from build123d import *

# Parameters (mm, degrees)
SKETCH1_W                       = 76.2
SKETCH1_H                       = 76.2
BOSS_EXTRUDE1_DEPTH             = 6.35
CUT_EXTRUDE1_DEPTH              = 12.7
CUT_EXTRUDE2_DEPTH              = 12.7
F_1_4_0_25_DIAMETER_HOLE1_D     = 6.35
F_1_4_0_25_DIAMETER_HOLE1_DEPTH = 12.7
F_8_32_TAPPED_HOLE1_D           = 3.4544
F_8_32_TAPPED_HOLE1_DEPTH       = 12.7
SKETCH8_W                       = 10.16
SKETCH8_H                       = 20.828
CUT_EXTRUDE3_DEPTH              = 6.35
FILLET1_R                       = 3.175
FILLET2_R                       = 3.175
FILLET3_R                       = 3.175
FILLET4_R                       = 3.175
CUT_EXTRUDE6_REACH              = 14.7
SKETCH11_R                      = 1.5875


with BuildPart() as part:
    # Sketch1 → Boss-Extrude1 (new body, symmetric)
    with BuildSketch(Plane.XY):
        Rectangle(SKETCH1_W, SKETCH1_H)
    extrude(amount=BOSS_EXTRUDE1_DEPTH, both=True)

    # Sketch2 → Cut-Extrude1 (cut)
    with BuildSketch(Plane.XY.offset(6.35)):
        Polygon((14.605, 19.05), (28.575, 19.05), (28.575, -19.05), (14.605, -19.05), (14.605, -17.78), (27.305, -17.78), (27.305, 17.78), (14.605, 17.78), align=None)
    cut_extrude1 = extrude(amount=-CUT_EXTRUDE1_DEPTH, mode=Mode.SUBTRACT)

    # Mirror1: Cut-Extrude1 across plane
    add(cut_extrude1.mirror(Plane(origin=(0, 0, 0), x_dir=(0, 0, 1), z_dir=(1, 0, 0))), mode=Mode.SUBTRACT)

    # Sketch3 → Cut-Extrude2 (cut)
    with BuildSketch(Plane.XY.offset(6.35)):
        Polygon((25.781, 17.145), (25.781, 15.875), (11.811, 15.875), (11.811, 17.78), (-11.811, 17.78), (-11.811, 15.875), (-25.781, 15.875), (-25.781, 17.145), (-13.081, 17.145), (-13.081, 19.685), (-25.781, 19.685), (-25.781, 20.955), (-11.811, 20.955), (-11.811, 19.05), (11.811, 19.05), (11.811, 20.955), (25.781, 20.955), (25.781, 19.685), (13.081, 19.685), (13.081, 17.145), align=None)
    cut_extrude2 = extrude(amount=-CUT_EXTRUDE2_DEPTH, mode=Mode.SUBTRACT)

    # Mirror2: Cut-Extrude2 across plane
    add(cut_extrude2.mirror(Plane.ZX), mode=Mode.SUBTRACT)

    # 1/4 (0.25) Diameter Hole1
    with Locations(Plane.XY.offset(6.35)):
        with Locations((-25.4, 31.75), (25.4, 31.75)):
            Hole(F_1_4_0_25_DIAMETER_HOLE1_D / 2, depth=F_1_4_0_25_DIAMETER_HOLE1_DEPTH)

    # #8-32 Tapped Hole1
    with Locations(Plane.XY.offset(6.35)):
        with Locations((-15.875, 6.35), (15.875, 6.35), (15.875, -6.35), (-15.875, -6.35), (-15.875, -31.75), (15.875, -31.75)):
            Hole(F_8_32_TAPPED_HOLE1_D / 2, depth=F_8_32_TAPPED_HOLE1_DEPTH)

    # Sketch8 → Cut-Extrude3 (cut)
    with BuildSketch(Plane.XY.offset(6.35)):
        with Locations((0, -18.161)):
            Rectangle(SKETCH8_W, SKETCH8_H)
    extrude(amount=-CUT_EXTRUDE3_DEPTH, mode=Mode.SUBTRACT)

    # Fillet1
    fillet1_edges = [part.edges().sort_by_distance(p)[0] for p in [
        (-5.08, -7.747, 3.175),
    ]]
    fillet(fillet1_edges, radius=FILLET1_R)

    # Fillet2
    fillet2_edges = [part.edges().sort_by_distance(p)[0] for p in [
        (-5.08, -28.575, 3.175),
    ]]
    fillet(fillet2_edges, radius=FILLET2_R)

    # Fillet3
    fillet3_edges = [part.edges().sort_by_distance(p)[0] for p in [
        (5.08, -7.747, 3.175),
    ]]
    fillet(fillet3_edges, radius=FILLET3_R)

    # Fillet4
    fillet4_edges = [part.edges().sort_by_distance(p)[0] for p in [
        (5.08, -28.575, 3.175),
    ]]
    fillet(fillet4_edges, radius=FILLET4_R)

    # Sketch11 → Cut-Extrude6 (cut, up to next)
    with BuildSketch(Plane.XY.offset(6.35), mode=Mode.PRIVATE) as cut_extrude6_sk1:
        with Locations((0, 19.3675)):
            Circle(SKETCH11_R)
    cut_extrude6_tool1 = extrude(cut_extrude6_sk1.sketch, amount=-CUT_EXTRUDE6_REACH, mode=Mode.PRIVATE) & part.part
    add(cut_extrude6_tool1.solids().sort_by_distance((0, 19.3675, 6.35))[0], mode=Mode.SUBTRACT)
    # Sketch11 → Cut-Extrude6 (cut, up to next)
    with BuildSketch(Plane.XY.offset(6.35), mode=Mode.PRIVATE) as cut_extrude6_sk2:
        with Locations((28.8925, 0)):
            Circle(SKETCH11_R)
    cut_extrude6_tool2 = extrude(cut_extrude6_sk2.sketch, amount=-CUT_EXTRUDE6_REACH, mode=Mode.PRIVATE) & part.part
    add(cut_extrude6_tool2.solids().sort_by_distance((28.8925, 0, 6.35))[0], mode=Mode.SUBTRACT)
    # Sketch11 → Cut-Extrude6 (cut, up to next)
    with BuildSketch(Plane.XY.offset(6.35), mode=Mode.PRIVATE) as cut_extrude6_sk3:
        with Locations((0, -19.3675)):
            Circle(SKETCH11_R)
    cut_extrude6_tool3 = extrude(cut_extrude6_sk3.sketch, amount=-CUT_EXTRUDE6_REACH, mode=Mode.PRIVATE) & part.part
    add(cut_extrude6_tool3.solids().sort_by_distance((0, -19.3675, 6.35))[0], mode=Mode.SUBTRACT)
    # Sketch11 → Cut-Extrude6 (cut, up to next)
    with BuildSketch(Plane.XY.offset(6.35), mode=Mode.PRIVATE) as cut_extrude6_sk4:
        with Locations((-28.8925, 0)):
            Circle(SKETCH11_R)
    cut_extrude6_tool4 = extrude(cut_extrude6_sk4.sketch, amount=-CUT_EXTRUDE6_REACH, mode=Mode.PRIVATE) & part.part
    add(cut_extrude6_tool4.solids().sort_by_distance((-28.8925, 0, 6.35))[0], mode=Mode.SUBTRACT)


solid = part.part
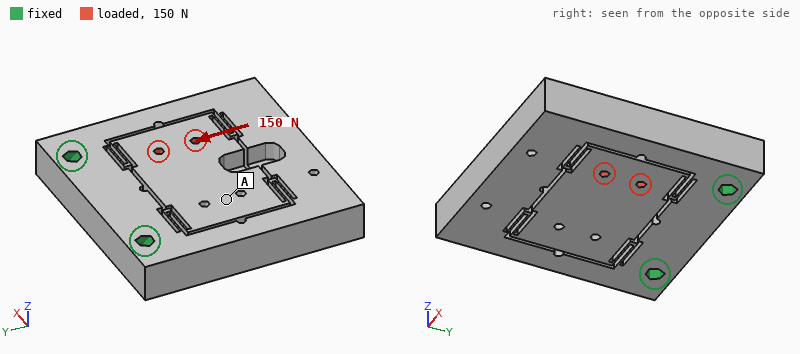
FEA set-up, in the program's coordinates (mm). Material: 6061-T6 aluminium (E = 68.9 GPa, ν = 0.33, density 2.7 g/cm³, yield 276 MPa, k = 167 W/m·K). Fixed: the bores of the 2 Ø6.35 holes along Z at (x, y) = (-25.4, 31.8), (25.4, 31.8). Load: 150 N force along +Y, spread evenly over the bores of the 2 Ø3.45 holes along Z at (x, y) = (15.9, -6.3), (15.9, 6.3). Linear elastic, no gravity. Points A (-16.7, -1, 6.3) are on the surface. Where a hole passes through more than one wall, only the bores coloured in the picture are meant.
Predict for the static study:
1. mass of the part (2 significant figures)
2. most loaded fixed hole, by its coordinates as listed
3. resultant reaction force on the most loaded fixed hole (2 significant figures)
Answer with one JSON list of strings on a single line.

["180 g", "(25.4, 31.8)", "110 N"]
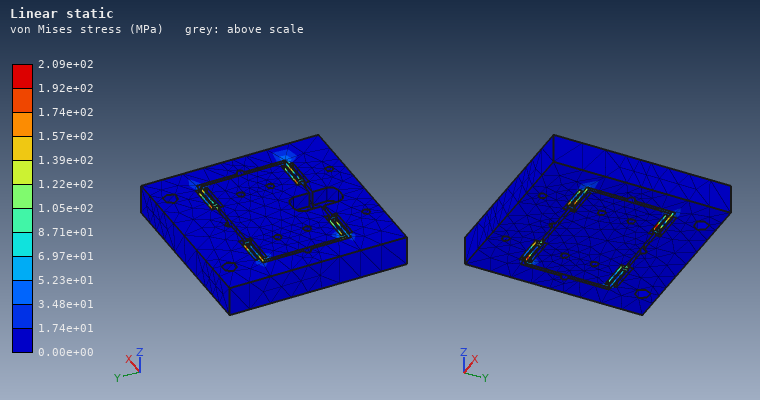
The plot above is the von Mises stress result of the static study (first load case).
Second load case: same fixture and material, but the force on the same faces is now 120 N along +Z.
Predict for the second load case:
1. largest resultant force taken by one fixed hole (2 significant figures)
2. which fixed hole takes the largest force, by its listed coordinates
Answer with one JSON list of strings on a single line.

["95 N", "(25.4, 31.8)"]
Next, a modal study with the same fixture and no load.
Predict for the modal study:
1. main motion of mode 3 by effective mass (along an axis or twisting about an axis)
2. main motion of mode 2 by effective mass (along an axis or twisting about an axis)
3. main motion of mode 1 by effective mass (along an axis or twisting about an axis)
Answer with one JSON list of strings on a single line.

["along X", "along Z", "along Y"]
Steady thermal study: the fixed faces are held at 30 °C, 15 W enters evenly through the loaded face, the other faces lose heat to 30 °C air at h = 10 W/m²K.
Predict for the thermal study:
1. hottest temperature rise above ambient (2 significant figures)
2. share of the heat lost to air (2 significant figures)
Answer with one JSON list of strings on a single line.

["60 K", "33 %"]
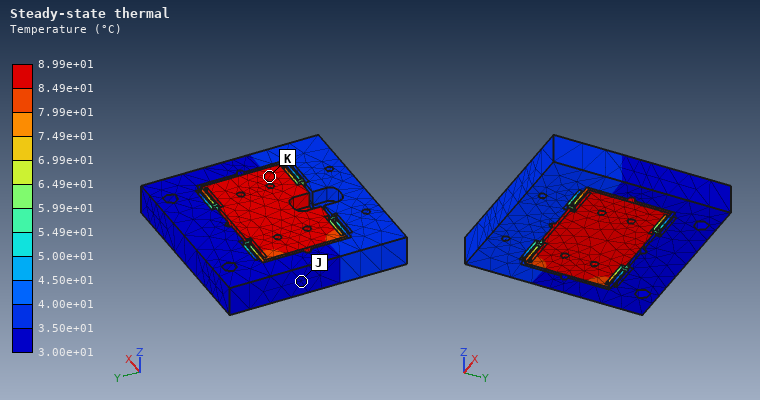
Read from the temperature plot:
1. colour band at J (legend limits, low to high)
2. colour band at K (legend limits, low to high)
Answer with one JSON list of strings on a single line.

["3.00e+01 to 3.50e+01 °C", "8.49e+01 to 8.99e+01 °C"]
